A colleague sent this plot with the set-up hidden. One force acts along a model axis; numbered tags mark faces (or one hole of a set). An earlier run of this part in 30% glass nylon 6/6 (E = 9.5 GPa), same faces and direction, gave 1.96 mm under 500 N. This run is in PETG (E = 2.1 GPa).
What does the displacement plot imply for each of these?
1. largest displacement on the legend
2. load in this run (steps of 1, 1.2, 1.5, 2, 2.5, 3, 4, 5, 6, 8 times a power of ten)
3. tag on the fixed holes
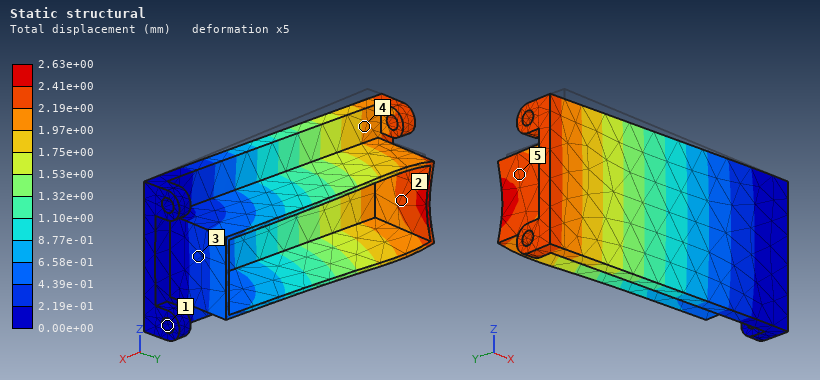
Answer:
2.63e+00 mm
150 N
1
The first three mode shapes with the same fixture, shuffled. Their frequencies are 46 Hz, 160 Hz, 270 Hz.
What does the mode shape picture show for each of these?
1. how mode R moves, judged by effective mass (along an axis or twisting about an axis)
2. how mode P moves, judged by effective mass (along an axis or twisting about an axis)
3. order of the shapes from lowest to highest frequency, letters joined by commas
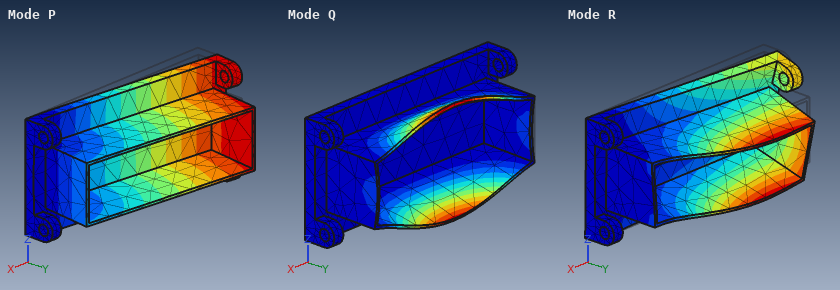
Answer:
along Z
along Y
P, R, Q
